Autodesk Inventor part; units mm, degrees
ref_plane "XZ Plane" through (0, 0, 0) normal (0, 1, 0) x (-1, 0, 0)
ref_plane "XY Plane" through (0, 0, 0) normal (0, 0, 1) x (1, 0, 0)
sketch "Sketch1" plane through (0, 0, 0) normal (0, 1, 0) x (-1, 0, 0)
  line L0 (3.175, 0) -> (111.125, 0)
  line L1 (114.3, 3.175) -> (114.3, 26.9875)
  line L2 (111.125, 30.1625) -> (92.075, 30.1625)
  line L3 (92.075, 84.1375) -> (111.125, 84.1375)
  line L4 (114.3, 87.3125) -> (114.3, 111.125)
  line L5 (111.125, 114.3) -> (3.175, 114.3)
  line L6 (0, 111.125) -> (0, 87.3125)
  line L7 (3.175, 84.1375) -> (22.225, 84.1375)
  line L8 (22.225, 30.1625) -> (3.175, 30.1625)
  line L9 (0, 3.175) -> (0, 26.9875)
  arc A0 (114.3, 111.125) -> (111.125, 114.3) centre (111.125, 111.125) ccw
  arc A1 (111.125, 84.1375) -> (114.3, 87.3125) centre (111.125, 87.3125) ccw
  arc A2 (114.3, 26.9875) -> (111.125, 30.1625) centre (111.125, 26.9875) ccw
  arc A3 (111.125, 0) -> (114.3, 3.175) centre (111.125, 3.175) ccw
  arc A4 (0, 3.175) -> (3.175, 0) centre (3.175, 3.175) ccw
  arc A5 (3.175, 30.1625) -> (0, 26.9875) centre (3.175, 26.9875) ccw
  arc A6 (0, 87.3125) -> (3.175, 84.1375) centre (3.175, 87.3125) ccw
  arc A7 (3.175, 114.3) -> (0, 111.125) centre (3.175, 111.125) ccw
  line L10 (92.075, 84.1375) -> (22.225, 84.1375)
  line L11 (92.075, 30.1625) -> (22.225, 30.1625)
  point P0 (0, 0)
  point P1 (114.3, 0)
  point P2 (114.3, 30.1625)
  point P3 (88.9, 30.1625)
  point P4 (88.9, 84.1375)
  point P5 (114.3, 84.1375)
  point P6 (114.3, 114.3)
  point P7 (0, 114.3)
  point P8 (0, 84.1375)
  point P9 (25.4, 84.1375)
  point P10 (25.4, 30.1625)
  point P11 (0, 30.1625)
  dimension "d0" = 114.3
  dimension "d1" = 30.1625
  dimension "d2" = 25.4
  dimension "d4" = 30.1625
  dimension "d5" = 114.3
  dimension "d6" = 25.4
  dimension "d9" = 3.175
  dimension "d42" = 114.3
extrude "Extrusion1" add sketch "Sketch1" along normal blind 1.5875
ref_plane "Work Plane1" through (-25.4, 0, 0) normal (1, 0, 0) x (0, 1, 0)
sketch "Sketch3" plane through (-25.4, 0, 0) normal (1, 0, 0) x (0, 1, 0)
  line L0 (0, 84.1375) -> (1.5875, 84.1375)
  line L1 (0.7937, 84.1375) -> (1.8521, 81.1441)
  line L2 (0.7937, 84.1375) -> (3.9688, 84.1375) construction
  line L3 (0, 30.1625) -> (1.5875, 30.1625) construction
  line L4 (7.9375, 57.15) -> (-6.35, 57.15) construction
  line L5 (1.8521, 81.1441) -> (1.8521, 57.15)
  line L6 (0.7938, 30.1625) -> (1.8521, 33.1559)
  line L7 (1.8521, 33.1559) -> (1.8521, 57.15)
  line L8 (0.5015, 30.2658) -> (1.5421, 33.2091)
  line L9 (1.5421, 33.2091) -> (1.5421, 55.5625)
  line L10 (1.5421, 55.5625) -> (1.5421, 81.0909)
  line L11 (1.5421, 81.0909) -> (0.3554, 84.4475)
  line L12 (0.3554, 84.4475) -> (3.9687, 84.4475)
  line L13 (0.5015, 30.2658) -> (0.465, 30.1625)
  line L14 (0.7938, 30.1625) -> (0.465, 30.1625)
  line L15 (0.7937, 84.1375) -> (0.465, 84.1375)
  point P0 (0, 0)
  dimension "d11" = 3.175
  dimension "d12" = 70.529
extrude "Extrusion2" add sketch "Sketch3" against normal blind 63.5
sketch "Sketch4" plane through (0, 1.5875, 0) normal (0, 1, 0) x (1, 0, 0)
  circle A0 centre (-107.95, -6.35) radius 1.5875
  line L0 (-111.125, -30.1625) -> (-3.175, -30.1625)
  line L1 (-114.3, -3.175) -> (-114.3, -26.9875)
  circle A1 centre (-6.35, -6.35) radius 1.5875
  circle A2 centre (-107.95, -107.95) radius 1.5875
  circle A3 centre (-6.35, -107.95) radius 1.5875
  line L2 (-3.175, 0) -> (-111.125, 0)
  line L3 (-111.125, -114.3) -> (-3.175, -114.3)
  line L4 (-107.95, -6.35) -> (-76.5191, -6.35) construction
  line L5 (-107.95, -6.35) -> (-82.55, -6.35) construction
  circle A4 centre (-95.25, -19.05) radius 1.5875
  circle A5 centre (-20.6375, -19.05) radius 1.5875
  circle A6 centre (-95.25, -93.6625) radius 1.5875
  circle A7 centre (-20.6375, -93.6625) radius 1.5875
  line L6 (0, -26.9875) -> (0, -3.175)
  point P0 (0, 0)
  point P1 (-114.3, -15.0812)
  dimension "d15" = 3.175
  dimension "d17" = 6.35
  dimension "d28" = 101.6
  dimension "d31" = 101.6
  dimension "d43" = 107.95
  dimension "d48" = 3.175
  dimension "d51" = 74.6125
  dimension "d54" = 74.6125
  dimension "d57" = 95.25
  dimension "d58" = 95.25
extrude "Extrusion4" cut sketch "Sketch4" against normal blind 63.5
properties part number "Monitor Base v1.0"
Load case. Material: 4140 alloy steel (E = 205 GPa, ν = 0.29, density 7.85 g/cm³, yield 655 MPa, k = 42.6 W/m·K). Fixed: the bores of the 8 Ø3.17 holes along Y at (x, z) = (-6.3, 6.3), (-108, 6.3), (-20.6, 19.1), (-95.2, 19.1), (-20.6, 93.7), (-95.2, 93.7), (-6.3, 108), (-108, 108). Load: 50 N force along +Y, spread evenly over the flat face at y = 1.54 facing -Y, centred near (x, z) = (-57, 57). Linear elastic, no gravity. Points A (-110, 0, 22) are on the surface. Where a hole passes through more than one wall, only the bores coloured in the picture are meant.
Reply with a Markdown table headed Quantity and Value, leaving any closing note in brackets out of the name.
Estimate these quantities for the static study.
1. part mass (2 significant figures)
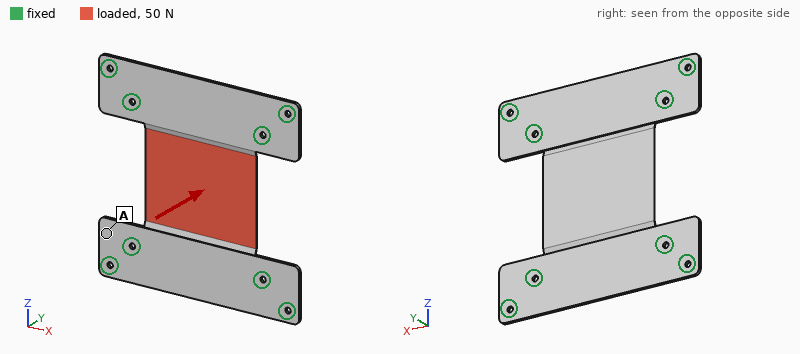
| Quantity | Value |
|---|---|
| part mass | 93 g |
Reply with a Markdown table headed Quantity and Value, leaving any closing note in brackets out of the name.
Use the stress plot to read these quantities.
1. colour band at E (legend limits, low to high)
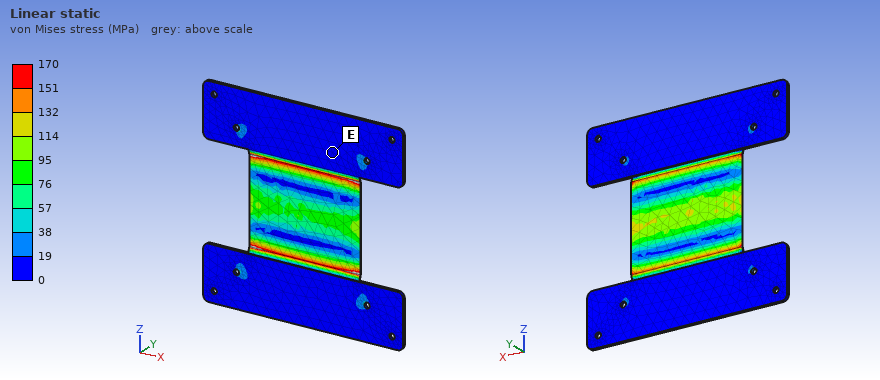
| Quantity | Value |
|---|---|
| colour band at E | 0 to 19 MPa |
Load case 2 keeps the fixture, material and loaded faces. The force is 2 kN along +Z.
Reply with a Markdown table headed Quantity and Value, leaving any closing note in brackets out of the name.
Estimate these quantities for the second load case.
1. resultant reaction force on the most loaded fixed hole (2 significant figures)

| Quantity | Value |
|---|---|
| resultant reaction force on the most loaded fixed hole | 600 N |
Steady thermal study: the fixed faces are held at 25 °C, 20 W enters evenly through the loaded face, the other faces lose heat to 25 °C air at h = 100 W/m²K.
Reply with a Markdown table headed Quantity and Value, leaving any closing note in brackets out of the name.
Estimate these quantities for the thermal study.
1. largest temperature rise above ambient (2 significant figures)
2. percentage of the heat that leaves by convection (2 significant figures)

| Quantity | Value |
|---|---|
| largest temperature rise above ambient | 55 K |
| percentage of the heat that leaves by convection | 92 % |
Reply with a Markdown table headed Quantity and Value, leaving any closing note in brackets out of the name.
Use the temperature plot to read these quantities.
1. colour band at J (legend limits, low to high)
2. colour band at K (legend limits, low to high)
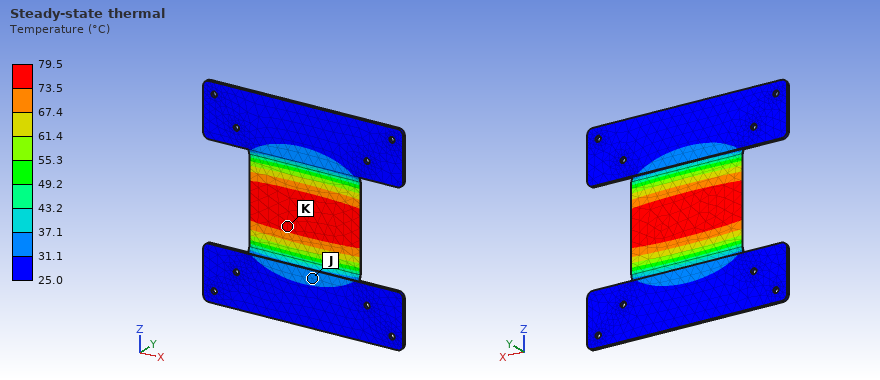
| Quantity | Value |
|---|---|
| colour band at J | 31.1 to 37.1 °C |
| colour band at K | 73.5 to 79.5 °C |
